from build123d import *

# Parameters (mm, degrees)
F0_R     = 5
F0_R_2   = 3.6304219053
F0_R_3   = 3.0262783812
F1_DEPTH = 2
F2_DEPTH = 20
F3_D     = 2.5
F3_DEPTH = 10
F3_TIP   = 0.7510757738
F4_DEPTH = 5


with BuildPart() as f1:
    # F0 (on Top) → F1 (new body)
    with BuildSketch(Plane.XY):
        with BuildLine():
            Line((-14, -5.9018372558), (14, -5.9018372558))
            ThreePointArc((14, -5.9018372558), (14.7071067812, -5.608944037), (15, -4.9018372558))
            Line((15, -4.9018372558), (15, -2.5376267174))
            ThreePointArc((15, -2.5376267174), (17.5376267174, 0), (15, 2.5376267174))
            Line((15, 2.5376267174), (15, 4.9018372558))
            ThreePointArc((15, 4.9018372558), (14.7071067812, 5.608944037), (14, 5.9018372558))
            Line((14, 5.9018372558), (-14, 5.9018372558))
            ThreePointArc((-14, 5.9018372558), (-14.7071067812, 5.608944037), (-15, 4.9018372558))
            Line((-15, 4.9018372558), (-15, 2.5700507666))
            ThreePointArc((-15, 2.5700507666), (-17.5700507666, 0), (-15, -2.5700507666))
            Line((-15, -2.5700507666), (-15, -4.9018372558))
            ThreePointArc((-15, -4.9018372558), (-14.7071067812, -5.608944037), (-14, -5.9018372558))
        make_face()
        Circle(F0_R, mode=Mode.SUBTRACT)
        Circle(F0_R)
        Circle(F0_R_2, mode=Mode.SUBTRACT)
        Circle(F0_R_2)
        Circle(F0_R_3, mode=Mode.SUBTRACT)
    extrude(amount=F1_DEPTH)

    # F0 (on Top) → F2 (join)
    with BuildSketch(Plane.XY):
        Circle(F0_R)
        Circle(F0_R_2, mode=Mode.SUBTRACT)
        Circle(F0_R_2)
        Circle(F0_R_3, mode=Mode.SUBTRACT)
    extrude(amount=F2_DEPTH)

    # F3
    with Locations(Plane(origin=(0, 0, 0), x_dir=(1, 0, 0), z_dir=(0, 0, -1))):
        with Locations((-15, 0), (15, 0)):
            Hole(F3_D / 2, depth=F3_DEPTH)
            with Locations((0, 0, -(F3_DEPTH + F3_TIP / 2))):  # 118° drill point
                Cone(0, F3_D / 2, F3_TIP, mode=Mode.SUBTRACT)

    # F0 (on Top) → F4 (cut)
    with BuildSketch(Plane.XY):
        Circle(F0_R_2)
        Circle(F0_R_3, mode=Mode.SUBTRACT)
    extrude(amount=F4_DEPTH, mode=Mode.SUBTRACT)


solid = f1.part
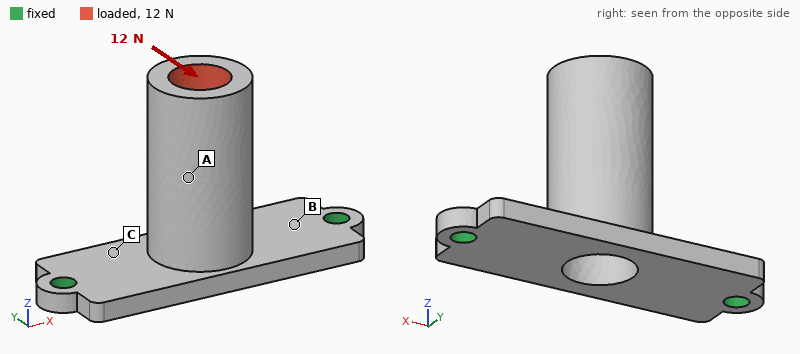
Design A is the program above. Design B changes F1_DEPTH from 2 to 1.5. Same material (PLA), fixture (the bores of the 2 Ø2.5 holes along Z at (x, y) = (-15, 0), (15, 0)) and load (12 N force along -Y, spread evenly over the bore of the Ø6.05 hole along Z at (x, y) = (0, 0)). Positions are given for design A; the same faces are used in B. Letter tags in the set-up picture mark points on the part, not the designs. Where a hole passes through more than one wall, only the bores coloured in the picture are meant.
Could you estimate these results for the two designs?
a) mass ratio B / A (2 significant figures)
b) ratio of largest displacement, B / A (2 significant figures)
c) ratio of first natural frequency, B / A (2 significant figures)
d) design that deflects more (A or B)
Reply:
0.91
2.2
0.68
B
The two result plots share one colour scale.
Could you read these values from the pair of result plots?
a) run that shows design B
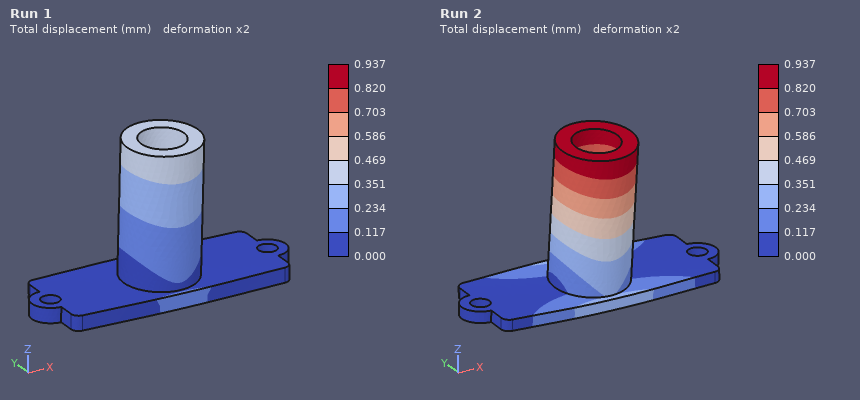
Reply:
Run 2
